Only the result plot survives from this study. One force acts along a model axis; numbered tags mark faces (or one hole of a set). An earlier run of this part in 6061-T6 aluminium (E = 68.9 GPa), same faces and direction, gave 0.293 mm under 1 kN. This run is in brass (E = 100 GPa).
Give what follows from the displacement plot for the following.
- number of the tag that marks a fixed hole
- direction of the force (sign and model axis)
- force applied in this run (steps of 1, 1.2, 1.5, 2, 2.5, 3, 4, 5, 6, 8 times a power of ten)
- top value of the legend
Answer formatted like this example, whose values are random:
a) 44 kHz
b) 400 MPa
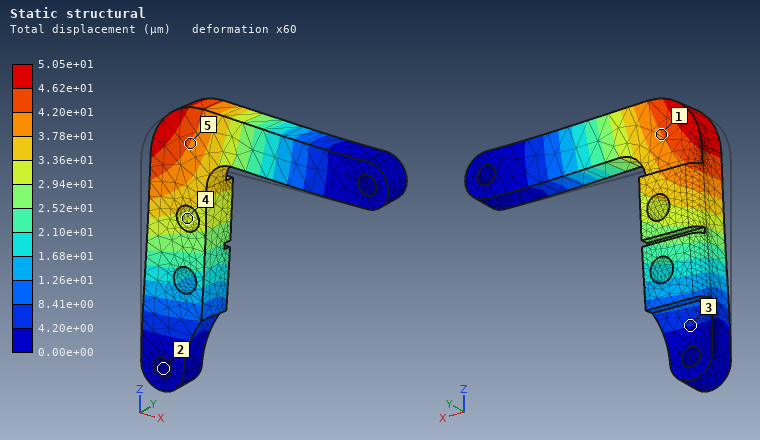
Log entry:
a) 2
b) +Y
c) 250 N
d) 5.05e+01 µm
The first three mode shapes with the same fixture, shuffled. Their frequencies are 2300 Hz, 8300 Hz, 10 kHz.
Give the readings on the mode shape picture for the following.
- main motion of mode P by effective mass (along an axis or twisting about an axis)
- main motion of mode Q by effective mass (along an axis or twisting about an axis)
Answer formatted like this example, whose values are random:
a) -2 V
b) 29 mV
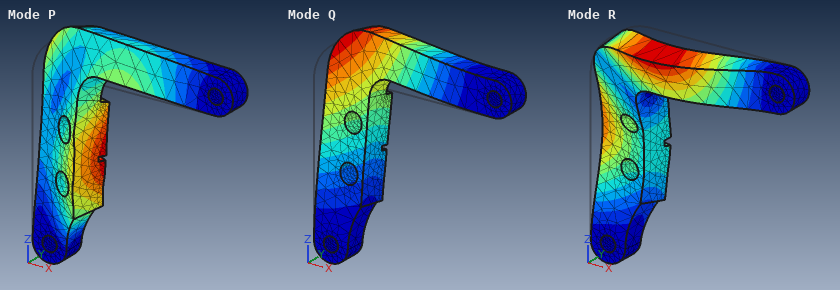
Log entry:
a) along X
b) along Y
